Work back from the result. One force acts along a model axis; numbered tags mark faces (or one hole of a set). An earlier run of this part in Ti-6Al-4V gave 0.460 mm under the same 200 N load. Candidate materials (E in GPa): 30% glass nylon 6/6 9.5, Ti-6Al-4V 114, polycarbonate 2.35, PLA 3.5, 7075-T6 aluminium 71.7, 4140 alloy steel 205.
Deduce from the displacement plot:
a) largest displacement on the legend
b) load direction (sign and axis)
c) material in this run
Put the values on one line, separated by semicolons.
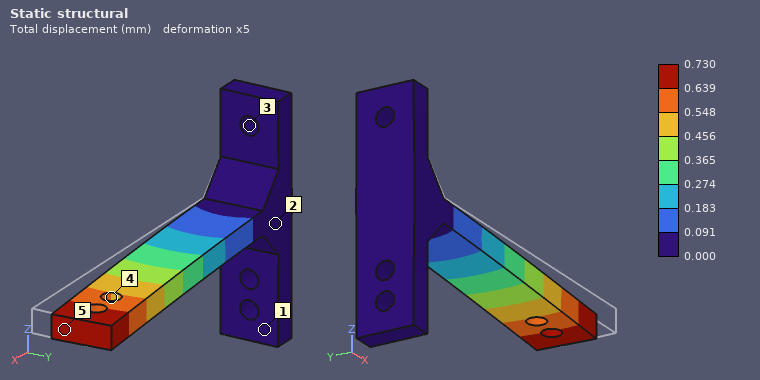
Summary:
0.730 mm; +Y; 7075-T6 aluminium
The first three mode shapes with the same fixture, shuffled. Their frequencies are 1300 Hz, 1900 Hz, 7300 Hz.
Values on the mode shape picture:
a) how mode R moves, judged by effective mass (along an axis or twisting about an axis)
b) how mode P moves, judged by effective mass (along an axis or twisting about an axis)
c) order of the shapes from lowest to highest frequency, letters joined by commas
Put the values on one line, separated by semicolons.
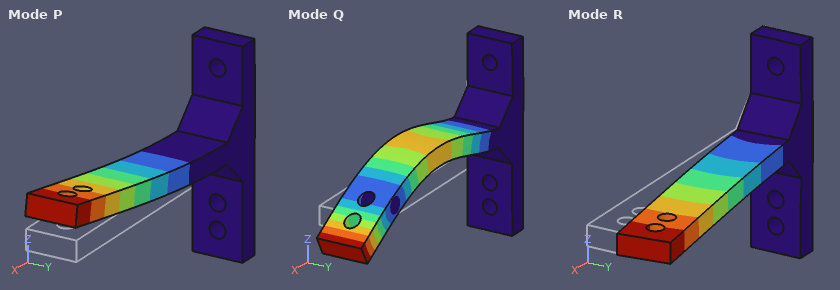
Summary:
along Y; along Z; P, R, Q
